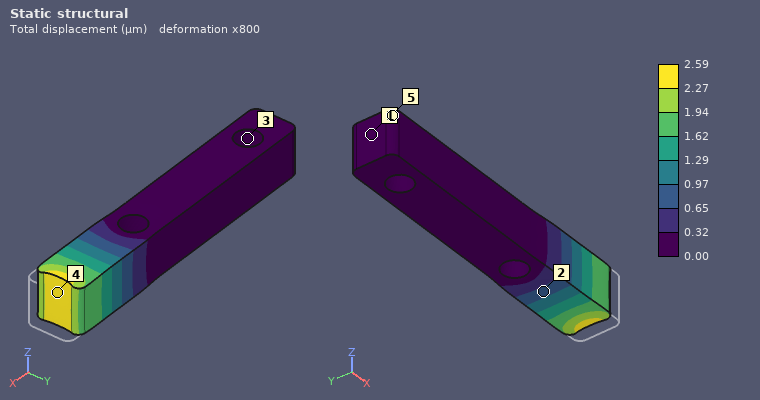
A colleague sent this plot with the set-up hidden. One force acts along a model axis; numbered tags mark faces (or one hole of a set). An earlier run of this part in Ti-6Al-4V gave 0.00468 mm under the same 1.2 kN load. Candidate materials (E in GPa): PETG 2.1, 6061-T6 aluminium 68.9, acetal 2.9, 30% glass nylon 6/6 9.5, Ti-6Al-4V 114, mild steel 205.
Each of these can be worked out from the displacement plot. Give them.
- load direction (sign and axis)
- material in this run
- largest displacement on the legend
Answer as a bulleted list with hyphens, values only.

- -X
- mild steel
- 2.59 µm
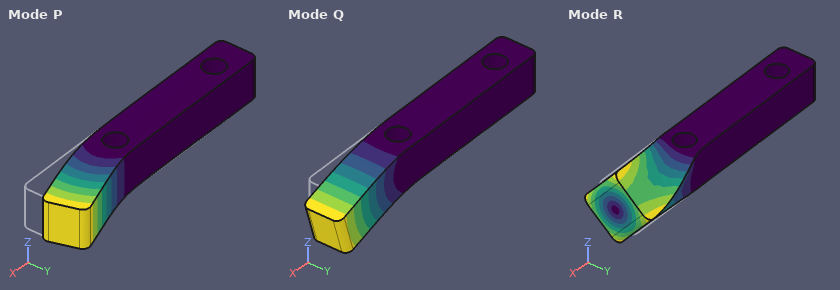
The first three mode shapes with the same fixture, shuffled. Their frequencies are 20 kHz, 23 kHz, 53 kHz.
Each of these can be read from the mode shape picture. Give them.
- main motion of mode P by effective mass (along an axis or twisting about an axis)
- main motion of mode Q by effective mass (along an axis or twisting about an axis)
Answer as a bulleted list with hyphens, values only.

- along Y
- along Z
